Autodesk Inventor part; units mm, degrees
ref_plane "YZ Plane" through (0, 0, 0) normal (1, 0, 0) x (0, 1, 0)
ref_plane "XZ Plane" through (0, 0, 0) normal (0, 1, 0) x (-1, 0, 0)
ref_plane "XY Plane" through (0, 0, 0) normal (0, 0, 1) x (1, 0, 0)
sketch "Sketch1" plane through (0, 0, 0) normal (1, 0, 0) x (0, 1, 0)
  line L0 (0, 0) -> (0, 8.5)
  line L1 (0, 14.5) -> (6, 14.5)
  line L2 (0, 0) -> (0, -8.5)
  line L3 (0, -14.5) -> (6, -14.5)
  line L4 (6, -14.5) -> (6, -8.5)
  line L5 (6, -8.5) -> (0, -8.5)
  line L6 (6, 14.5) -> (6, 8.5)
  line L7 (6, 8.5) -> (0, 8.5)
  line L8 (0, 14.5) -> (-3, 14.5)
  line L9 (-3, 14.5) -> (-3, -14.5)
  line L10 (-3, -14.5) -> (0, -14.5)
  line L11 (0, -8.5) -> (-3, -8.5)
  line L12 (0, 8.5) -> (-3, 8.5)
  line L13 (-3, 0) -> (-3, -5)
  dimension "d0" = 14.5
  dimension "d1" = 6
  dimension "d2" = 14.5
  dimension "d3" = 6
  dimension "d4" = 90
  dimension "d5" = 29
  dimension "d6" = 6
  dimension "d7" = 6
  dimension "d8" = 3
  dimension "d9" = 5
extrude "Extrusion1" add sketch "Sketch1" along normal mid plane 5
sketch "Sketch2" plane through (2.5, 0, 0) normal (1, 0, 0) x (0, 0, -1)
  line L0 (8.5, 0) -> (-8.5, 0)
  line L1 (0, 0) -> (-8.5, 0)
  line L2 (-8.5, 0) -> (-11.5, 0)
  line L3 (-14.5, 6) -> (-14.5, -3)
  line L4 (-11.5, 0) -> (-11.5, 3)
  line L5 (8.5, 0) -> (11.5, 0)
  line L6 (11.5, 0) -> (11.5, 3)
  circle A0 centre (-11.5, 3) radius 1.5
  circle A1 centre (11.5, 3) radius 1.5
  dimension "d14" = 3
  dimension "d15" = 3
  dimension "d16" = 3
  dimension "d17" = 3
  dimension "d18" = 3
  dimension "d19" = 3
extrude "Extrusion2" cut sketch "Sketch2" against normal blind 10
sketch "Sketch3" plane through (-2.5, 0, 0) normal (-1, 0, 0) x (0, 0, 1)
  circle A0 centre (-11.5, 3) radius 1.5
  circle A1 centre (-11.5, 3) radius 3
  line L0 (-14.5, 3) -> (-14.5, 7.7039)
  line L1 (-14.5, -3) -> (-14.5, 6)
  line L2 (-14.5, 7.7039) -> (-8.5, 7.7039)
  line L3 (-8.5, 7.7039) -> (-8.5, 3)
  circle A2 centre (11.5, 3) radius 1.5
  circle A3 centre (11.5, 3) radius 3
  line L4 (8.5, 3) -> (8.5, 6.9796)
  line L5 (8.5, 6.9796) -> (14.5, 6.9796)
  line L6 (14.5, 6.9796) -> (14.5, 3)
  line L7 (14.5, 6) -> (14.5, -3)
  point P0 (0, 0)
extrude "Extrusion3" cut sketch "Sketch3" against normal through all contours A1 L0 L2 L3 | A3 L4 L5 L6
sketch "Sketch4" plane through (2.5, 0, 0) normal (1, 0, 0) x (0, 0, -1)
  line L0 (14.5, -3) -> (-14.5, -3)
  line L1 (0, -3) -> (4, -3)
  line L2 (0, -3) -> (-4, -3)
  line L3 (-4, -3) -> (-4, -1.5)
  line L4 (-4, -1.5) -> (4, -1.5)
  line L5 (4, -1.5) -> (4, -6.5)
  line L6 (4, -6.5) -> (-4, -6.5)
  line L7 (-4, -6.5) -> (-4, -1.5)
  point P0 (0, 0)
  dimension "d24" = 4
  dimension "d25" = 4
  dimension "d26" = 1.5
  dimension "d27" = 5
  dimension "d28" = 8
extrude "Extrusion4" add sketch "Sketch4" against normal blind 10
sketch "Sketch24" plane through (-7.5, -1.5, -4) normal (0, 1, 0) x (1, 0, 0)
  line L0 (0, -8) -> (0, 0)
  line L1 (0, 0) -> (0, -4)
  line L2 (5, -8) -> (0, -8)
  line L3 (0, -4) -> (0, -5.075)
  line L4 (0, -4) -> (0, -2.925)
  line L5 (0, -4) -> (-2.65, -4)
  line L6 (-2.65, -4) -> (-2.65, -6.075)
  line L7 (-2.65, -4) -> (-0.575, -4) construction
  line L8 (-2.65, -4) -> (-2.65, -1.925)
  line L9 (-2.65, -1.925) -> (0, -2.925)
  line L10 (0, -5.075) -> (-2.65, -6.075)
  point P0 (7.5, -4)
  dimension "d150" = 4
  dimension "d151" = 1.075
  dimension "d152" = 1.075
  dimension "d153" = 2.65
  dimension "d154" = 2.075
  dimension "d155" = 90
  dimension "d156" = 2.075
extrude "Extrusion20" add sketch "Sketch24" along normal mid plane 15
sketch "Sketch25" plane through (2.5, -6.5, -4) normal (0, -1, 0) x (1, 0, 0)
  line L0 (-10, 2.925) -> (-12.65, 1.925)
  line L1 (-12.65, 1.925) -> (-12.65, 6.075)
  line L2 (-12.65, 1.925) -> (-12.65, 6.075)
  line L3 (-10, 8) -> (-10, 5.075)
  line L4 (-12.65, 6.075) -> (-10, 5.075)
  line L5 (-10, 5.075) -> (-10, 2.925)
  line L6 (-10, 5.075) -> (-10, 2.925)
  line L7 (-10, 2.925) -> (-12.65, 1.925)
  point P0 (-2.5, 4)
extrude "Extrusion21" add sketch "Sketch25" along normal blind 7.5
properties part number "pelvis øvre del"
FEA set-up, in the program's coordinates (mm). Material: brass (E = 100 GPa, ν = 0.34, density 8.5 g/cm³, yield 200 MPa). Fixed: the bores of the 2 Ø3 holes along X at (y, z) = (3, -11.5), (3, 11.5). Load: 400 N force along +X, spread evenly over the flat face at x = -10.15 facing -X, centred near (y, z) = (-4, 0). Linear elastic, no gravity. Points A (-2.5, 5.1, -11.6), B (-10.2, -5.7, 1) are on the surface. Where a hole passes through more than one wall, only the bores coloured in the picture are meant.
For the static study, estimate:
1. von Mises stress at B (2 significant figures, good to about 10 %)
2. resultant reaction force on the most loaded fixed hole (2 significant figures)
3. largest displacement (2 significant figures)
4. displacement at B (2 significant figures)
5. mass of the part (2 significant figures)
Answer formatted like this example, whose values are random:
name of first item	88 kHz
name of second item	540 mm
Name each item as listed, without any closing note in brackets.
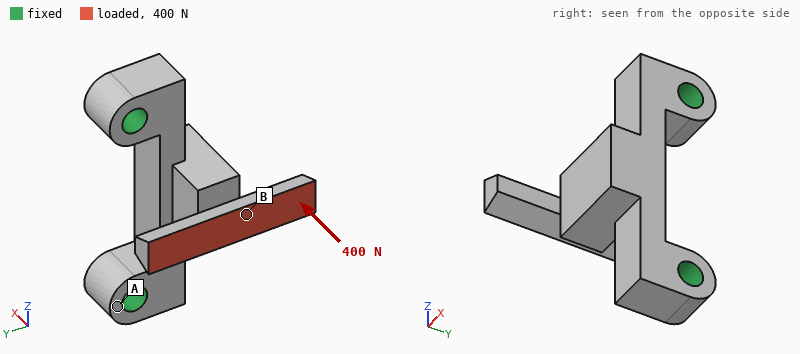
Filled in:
von Mises stress at B	100 MPa
resultant reaction force on the most loaded fixed hole	200 N
largest displacement	95 µm
displacement at B	45 µm
mass of the part	10 g
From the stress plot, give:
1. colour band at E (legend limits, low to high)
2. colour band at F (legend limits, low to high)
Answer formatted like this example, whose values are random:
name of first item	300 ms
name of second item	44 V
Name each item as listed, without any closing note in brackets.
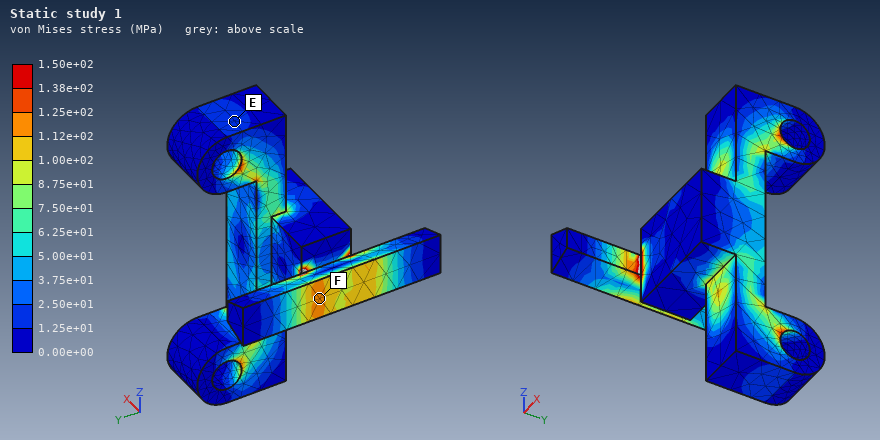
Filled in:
colour band at E	1.25e+01 to 2.50e+01 MPa
colour band at F	1.12e+02 to 1.25e+02 MPa
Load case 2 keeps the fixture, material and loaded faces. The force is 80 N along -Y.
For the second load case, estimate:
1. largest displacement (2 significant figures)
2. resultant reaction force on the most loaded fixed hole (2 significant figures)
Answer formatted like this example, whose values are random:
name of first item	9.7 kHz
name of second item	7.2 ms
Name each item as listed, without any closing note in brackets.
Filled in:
largest displacement	51 µm
resultant reaction force on the most loaded fixed hole	56 N
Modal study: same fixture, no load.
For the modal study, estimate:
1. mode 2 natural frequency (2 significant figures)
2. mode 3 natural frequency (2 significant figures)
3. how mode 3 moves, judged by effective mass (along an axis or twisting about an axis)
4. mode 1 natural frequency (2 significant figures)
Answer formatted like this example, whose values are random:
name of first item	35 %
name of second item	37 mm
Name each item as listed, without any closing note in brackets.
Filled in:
mode 2 natural frequency	12 kHz
mode 3 natural frequency	13 kHz
how mode 3 moves, judged by effective mass	along X
mode 1 natural frequency	5200 Hz
